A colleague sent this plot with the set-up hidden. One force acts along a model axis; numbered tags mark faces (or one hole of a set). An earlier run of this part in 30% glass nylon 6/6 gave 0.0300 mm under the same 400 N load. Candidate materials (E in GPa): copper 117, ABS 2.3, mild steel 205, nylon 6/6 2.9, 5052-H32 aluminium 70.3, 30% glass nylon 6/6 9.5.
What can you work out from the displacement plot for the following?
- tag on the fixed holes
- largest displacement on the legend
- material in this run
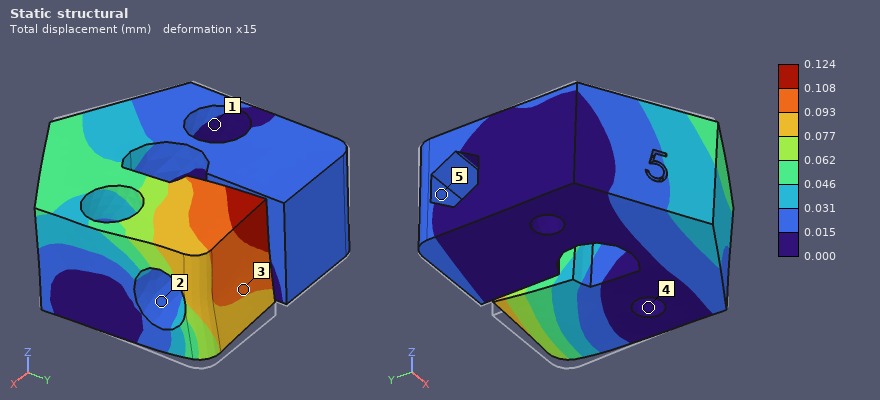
4
0.124 mm
ABS
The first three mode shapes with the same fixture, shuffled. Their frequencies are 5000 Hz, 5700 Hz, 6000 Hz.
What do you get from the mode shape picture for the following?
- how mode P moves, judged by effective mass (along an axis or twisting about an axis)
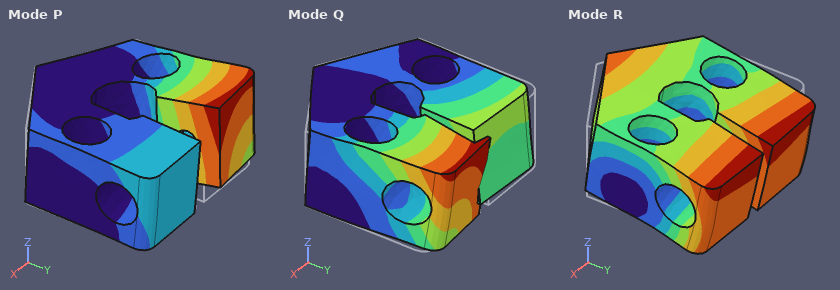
along X
